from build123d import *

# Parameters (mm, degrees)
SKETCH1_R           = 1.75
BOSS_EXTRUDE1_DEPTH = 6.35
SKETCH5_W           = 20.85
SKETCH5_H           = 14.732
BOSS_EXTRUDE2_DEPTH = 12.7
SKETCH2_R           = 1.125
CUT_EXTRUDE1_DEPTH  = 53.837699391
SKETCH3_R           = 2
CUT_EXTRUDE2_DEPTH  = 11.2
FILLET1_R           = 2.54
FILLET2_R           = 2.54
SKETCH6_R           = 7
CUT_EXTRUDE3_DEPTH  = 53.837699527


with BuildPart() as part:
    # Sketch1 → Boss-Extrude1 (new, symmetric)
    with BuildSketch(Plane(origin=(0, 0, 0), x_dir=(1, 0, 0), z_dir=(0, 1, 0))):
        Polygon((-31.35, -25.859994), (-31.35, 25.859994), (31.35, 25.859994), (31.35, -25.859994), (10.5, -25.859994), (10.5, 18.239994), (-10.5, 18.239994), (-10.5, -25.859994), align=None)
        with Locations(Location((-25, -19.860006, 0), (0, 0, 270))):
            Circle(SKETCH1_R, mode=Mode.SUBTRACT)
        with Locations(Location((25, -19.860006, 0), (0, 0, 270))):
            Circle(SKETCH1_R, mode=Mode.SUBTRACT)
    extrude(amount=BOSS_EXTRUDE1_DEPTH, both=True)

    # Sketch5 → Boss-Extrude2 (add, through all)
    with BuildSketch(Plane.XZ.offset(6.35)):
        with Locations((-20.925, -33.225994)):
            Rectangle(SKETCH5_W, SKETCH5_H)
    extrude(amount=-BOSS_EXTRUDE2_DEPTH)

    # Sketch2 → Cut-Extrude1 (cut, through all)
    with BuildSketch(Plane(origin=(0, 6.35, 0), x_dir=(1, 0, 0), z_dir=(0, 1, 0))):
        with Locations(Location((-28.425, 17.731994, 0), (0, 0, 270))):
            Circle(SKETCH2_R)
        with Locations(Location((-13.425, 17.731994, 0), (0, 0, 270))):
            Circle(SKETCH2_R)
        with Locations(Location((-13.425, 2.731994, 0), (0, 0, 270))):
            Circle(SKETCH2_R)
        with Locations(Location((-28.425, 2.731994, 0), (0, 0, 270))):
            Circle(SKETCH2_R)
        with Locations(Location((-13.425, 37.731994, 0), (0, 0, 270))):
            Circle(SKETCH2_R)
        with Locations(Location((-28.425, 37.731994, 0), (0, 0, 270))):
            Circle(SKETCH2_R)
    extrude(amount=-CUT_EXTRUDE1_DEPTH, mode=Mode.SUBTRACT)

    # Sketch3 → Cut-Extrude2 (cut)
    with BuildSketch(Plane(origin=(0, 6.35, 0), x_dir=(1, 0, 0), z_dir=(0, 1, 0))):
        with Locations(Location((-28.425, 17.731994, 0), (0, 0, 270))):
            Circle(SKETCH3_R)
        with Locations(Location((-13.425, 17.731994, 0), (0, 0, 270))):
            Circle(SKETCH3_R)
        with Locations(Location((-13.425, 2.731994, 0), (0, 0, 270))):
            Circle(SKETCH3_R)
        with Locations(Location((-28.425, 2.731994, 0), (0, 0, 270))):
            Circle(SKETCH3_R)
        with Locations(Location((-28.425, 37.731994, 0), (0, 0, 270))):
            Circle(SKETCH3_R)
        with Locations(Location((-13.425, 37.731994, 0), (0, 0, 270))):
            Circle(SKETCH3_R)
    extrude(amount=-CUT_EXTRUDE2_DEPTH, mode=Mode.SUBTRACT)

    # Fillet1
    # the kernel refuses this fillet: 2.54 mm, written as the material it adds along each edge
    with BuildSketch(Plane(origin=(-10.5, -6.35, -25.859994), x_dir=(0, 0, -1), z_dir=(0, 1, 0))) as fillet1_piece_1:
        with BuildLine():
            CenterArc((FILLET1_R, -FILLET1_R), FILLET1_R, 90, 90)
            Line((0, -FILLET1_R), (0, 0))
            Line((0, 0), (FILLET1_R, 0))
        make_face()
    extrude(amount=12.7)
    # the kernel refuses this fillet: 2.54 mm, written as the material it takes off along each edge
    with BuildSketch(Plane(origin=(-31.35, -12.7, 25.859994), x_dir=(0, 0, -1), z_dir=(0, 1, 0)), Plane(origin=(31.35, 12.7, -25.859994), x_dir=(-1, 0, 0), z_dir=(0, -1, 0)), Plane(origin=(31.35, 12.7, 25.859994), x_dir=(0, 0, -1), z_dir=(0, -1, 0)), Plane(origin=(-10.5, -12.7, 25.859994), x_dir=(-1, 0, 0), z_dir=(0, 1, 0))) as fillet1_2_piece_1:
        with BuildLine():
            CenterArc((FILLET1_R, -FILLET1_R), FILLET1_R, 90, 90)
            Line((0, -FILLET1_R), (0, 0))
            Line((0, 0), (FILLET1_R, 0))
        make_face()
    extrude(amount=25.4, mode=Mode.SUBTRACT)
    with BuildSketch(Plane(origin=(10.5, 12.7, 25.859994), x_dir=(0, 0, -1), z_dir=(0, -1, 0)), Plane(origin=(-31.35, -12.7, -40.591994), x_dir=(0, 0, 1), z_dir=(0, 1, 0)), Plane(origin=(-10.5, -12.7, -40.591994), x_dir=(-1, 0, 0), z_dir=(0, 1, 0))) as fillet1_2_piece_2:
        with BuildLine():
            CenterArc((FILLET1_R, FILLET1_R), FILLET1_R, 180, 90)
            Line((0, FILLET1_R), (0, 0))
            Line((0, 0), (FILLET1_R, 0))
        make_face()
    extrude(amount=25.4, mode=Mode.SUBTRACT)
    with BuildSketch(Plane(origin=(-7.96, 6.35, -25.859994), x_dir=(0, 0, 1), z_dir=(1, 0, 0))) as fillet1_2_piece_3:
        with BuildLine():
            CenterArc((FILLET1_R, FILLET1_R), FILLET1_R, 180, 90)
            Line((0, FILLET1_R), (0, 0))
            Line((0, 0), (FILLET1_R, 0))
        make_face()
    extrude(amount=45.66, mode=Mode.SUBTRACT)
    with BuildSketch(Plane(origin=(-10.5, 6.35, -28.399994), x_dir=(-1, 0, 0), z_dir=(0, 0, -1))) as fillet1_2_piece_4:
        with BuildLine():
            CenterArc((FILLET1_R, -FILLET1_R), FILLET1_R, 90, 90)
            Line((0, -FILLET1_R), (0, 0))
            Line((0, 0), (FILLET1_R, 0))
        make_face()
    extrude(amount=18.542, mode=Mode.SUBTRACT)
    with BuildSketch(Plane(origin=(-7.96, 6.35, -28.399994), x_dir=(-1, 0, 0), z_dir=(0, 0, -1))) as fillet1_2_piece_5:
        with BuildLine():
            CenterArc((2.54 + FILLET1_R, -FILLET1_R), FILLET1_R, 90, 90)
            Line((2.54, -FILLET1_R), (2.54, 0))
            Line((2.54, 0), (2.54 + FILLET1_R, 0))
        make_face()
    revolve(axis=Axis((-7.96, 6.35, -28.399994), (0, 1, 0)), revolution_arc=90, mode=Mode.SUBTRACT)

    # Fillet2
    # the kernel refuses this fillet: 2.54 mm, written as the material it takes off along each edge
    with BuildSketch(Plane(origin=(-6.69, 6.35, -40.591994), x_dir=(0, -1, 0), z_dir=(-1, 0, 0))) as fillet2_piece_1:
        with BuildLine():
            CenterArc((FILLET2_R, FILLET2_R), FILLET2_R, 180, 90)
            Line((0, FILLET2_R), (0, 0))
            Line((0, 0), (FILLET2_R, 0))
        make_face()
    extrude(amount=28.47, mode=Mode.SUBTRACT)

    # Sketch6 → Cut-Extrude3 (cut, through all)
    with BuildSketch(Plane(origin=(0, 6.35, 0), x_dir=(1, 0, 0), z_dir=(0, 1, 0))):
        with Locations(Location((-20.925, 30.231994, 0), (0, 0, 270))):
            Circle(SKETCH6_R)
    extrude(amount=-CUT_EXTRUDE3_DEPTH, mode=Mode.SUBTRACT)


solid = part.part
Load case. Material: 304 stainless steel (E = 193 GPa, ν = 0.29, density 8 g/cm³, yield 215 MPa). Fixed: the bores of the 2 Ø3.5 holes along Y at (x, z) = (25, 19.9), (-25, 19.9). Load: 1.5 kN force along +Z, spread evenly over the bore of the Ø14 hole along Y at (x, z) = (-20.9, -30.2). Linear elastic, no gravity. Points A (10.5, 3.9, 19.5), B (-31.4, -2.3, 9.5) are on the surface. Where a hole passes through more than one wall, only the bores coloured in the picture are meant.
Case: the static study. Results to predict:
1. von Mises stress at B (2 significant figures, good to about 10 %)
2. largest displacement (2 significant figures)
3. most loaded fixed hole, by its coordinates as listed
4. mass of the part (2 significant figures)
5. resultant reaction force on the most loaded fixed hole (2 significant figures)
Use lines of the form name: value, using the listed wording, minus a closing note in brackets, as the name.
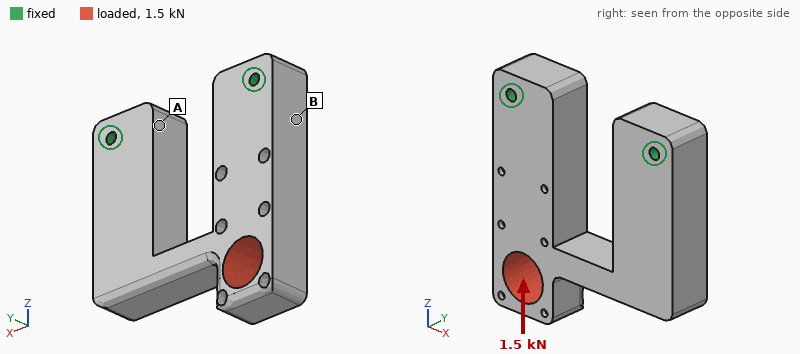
von Mises stress at B: 7.9 MPa
largest displacement: 4.0 µm
most loaded fixed hole, by its coordinates as listed: (-25, 19.9)
mass of the part: 240 g
resultant reaction force on the most loaded fixed hole: 1.4 kN
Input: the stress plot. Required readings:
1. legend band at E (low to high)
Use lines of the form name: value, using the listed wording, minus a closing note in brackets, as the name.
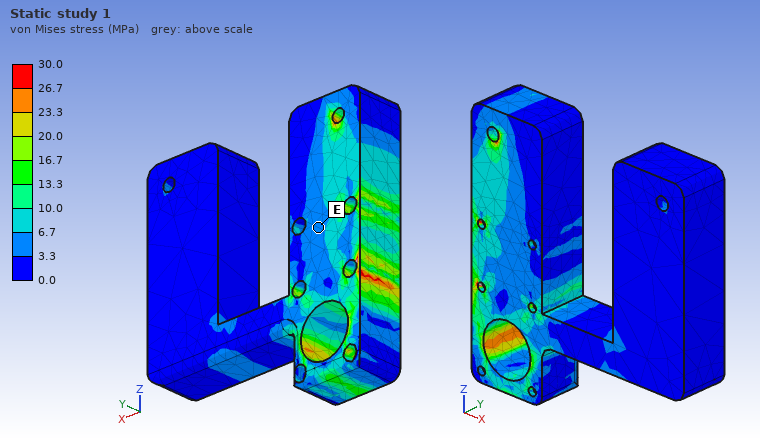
legend band at E: 3.3 to 6.7 MPa
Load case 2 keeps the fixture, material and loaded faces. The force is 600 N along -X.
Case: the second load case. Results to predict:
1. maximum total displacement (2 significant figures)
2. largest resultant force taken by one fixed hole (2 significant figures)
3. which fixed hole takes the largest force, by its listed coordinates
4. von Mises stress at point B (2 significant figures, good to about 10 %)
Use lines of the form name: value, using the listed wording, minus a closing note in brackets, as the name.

maximum total displacement: 15 µm
largest resultant force taken by one fixed hole: 510 N
which fixed hole takes the largest force, by its listed coordinates: (25, 19.9)
von Mises stress at point B: 6.8 MPa
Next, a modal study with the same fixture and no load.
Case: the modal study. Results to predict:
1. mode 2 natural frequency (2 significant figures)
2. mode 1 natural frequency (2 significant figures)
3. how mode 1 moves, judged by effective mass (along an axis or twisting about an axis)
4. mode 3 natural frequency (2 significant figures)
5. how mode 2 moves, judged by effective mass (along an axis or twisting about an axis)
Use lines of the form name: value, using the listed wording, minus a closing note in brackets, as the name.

mode 2 natural frequency: 4100 Hz
mode 1 natural frequency: 3000 Hz
how mode 1 moves, judged by effective mass: along Y
mode 3 natural frequency: 5400 Hz
how mode 2 moves, judged by effective mass: along X
